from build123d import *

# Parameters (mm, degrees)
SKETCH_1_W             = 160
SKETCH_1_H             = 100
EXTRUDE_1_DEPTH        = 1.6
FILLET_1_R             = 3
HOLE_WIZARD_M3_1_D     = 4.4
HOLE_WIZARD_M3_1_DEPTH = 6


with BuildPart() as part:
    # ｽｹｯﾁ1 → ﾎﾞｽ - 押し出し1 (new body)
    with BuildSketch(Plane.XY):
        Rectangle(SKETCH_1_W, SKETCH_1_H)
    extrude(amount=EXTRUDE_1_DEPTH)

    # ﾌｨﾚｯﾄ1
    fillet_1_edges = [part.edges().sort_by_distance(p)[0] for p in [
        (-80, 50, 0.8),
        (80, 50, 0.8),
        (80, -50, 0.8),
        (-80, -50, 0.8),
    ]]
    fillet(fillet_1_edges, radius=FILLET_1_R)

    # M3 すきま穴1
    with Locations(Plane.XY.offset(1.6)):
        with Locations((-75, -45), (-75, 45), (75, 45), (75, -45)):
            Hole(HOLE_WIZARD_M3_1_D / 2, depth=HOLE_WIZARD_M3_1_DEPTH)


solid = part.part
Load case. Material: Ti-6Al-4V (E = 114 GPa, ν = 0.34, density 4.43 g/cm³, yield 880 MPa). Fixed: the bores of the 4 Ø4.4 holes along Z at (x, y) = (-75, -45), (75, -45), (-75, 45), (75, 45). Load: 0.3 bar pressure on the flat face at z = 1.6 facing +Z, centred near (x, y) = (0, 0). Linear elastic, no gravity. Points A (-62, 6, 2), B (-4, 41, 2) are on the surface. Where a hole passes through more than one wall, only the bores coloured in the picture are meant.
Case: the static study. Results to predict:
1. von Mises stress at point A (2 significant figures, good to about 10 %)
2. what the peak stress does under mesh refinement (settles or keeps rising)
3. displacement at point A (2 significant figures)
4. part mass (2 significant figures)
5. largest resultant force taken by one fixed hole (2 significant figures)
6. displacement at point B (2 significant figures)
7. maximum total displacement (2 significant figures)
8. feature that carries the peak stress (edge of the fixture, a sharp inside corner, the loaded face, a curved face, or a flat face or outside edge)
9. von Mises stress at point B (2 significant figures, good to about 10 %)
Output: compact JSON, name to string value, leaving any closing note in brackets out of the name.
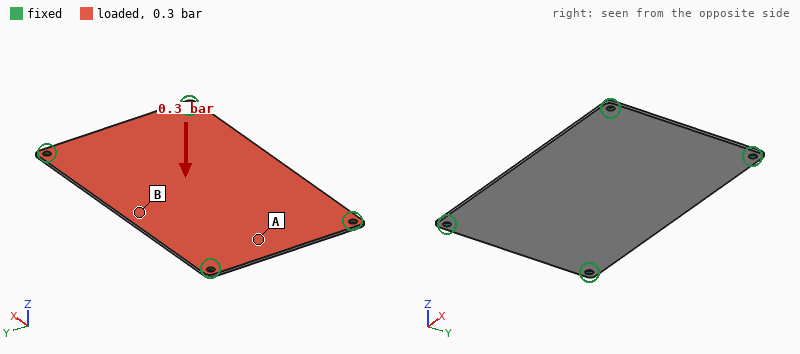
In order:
{"von Mises stress at point A": "39 MPa", "what the peak stress does under mesh refinement": "keeps rising", "displacement at point A": "0.47 mm", "part mass": "110 g", "largest resultant force taken by one fixed hole": "120 N", "displacement at point B": "1.5 mm", "maximum total displacement": "1.6 mm", "feature that carries the peak stress": "edge of the fixture", "von Mises stress at point B": "85 MPa"}
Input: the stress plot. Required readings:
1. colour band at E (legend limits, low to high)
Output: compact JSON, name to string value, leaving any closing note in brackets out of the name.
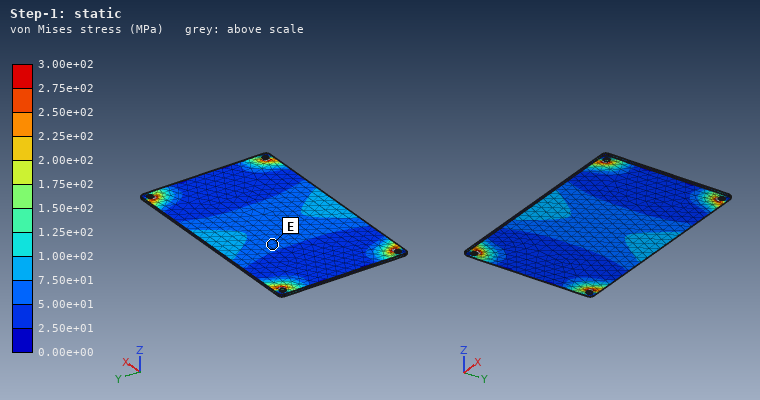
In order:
{"colour band at E": "5.00e+01 to 7.50e+01 MPa"}
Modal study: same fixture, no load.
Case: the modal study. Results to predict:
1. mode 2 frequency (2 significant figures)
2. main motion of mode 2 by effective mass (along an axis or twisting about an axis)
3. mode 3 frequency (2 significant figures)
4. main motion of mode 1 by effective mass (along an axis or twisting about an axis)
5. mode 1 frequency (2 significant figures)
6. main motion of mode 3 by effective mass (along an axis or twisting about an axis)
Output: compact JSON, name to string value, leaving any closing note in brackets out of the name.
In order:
{"mode 2 frequency": "520 Hz", "main motion of mode 2 by effective mass": "twisting about X", "mode 3 frequency": "790 Hz", "main motion of mode 1 by effective mass": "along Z", "mode 1 frequency": "300 Hz", "main motion of mode 3 by effective mass": "twisting about Y"}
